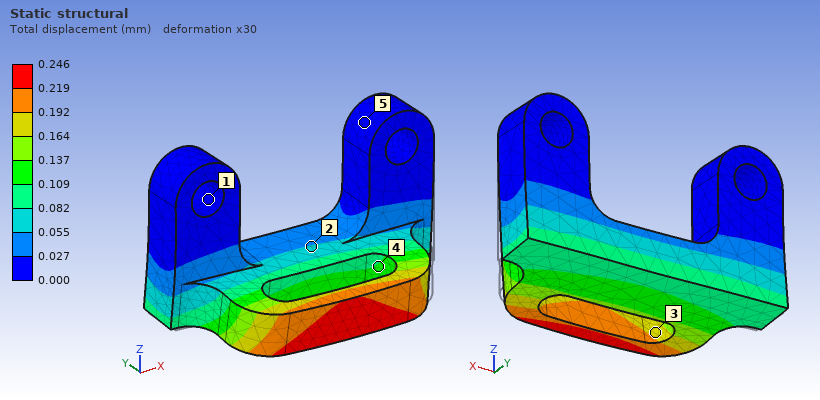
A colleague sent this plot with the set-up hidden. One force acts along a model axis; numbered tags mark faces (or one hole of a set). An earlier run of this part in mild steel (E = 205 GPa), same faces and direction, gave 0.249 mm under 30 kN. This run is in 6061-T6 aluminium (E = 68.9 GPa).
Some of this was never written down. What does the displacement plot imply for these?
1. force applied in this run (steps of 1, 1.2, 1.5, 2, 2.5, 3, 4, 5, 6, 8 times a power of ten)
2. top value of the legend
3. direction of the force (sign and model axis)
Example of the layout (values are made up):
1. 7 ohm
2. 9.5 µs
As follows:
1. 10 kN
2. 0.246 mm
3. -Z
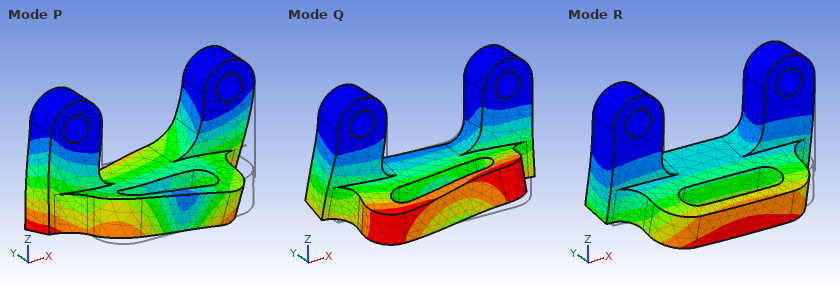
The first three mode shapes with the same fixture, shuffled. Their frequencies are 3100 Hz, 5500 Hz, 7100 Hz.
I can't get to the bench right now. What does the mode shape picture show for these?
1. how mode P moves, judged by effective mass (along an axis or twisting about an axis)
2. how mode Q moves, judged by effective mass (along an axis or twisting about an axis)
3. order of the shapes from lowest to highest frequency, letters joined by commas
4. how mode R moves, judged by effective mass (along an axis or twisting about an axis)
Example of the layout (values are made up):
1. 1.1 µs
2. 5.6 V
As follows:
1. along X
2. along X
3. R, Q, P
4. along Y
